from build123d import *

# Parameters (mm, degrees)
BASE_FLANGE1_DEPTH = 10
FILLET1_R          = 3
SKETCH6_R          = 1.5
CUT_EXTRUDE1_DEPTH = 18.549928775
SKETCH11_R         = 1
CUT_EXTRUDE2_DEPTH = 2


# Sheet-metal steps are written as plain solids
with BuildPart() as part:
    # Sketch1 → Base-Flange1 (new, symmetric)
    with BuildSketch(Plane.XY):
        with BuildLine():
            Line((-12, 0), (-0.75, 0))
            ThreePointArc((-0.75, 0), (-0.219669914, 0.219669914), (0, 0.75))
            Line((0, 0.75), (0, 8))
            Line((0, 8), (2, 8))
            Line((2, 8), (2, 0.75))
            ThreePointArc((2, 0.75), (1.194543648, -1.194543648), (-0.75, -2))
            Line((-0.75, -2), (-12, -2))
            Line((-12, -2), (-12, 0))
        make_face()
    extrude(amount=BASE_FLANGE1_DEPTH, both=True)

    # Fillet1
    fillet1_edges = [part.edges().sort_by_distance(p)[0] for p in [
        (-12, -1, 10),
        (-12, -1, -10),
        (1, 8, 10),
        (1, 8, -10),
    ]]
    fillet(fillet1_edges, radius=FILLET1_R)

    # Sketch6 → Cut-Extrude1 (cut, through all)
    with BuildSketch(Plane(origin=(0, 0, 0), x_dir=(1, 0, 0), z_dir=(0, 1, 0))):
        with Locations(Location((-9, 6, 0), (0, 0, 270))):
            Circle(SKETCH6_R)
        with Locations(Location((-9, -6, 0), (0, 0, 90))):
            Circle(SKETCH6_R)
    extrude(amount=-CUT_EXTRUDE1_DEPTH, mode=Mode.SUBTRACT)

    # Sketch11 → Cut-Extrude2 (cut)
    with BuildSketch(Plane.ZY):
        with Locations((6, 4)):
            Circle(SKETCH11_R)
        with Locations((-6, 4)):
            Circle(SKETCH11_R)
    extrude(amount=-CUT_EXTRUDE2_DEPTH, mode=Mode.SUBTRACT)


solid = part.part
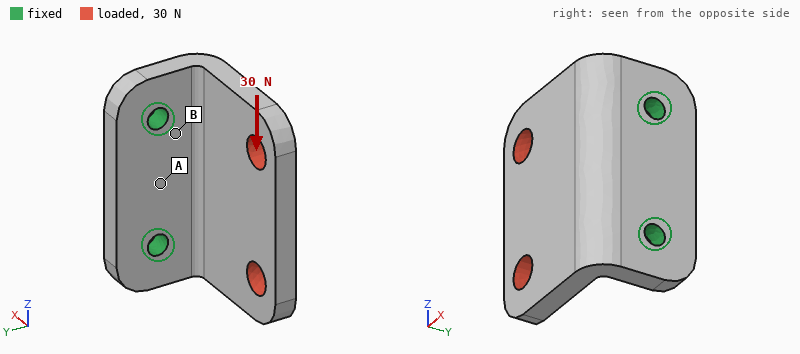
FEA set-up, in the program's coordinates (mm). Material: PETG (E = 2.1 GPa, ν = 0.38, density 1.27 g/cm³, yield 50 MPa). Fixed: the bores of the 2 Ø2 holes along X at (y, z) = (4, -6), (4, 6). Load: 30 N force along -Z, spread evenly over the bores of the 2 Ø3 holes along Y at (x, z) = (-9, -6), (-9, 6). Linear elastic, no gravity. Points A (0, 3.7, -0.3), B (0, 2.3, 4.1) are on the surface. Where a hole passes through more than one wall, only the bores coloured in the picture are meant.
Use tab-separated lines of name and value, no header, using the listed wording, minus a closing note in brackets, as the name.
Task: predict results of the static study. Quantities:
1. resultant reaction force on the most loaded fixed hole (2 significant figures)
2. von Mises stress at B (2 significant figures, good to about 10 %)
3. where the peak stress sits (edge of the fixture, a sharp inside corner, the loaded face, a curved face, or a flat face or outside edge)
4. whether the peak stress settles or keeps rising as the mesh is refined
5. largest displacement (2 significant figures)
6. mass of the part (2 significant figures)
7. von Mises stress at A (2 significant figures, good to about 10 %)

resultant reaction force on the most loaded fixed hole	29 N
von Mises stress at B	6.2 MPa
where the peak stress sits	edge of the fixture
whether the peak stress settles or keeps rising as the mesh is refined	keeps rising
largest displacement	0.15 mm
mass of the part	1.0 g
von Mises stress at A	2.7 MPa
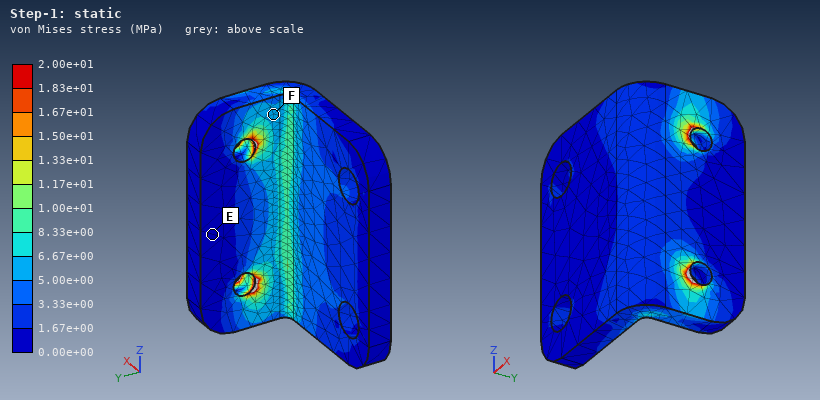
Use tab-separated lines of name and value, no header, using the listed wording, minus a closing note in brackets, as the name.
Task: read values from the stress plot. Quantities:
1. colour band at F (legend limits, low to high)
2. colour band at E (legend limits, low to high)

colour band at F	5.00e+00 to 6.67e+00 MPa
colour band at E	0.00e+00 to 1.67e+00 MPa
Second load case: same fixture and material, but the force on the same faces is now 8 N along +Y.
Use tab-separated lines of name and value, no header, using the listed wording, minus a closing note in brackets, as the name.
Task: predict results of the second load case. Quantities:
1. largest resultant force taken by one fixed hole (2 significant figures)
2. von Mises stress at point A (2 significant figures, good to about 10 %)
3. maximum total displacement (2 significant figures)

largest resultant force taken by one fixed hole	4.1 N
von Mises stress at point A	2.6 MPa
maximum total displacement	0.28 mm
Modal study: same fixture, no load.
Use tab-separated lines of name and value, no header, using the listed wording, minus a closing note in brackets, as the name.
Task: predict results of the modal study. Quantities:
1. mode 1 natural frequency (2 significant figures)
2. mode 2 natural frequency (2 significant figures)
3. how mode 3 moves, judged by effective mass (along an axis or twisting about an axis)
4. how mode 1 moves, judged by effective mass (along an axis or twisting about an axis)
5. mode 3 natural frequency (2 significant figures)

mode 1 natural frequency	1700 Hz
mode 2 natural frequency	3400 Hz
how mode 3 moves, judged by effective mass	along Z
how mode 1 moves, judged by effective mass	along Y
mode 3 natural frequency	5300 Hz
